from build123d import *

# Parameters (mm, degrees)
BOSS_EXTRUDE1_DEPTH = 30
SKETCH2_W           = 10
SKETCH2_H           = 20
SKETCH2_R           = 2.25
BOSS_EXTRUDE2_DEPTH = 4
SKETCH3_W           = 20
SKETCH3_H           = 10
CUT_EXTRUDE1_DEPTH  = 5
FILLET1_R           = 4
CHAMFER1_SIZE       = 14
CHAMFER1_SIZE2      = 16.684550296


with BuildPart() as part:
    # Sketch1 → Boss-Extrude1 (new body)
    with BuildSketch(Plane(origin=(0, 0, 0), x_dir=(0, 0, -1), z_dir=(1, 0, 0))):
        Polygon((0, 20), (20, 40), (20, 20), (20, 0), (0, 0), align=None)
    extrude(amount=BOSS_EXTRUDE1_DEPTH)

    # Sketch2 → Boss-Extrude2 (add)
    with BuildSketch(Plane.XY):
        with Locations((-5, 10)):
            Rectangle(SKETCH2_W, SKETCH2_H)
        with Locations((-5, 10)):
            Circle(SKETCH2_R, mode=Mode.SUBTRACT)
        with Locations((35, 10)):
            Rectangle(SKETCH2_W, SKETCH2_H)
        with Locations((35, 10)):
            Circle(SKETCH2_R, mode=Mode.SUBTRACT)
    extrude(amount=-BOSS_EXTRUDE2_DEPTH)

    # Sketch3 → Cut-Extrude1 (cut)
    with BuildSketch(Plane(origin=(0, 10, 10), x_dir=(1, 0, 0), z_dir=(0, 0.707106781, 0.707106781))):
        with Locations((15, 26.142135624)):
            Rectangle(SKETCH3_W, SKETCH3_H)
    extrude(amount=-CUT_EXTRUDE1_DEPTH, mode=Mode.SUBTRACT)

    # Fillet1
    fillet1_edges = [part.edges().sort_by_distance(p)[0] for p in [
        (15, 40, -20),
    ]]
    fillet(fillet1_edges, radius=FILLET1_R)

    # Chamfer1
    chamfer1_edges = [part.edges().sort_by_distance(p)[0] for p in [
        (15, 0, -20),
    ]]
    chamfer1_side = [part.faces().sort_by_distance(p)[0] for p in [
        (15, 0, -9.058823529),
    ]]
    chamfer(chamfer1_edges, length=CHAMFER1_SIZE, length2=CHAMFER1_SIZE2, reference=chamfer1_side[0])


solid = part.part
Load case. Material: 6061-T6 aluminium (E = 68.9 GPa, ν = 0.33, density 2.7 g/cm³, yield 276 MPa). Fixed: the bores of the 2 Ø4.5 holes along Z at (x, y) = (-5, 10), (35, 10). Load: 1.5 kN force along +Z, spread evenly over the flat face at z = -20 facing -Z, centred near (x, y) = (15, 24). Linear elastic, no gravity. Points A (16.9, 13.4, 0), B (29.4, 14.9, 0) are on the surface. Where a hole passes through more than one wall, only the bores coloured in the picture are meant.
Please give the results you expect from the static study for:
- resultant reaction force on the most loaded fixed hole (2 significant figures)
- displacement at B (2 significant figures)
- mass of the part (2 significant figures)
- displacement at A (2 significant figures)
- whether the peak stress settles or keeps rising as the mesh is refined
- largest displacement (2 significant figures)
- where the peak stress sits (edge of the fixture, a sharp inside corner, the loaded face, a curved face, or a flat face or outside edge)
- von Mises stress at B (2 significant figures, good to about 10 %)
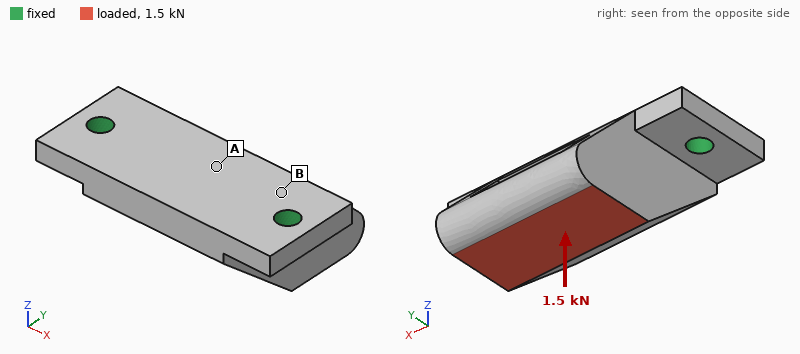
840 N
0.026 mm
39 g
0.024 mm
keeps rising
0.15 mm
edge of the fixture
63 MPa
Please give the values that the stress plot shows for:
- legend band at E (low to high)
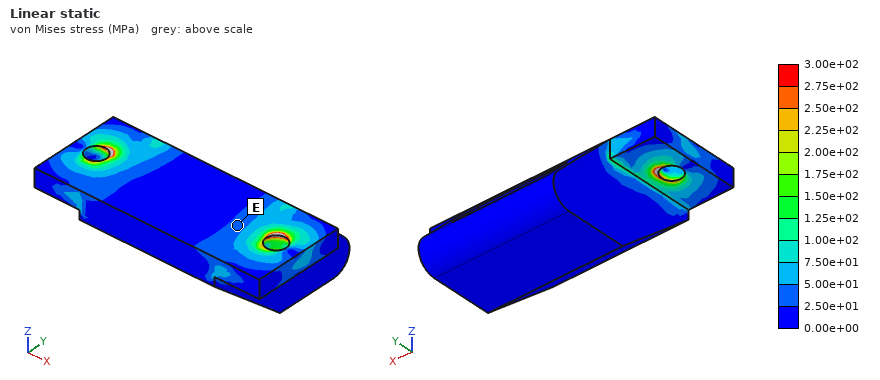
2.50e+01 to 5.00e+01 MPa
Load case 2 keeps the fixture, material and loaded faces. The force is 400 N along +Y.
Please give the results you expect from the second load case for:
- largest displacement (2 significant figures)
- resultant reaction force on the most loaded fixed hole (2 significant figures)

51 µm
200 N
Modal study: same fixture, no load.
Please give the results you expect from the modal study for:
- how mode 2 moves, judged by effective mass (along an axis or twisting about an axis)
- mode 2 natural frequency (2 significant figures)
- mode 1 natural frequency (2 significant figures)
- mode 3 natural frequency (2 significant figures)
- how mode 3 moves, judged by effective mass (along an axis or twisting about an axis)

along Z
13 kHz
3800 Hz
14 kHz
along X
